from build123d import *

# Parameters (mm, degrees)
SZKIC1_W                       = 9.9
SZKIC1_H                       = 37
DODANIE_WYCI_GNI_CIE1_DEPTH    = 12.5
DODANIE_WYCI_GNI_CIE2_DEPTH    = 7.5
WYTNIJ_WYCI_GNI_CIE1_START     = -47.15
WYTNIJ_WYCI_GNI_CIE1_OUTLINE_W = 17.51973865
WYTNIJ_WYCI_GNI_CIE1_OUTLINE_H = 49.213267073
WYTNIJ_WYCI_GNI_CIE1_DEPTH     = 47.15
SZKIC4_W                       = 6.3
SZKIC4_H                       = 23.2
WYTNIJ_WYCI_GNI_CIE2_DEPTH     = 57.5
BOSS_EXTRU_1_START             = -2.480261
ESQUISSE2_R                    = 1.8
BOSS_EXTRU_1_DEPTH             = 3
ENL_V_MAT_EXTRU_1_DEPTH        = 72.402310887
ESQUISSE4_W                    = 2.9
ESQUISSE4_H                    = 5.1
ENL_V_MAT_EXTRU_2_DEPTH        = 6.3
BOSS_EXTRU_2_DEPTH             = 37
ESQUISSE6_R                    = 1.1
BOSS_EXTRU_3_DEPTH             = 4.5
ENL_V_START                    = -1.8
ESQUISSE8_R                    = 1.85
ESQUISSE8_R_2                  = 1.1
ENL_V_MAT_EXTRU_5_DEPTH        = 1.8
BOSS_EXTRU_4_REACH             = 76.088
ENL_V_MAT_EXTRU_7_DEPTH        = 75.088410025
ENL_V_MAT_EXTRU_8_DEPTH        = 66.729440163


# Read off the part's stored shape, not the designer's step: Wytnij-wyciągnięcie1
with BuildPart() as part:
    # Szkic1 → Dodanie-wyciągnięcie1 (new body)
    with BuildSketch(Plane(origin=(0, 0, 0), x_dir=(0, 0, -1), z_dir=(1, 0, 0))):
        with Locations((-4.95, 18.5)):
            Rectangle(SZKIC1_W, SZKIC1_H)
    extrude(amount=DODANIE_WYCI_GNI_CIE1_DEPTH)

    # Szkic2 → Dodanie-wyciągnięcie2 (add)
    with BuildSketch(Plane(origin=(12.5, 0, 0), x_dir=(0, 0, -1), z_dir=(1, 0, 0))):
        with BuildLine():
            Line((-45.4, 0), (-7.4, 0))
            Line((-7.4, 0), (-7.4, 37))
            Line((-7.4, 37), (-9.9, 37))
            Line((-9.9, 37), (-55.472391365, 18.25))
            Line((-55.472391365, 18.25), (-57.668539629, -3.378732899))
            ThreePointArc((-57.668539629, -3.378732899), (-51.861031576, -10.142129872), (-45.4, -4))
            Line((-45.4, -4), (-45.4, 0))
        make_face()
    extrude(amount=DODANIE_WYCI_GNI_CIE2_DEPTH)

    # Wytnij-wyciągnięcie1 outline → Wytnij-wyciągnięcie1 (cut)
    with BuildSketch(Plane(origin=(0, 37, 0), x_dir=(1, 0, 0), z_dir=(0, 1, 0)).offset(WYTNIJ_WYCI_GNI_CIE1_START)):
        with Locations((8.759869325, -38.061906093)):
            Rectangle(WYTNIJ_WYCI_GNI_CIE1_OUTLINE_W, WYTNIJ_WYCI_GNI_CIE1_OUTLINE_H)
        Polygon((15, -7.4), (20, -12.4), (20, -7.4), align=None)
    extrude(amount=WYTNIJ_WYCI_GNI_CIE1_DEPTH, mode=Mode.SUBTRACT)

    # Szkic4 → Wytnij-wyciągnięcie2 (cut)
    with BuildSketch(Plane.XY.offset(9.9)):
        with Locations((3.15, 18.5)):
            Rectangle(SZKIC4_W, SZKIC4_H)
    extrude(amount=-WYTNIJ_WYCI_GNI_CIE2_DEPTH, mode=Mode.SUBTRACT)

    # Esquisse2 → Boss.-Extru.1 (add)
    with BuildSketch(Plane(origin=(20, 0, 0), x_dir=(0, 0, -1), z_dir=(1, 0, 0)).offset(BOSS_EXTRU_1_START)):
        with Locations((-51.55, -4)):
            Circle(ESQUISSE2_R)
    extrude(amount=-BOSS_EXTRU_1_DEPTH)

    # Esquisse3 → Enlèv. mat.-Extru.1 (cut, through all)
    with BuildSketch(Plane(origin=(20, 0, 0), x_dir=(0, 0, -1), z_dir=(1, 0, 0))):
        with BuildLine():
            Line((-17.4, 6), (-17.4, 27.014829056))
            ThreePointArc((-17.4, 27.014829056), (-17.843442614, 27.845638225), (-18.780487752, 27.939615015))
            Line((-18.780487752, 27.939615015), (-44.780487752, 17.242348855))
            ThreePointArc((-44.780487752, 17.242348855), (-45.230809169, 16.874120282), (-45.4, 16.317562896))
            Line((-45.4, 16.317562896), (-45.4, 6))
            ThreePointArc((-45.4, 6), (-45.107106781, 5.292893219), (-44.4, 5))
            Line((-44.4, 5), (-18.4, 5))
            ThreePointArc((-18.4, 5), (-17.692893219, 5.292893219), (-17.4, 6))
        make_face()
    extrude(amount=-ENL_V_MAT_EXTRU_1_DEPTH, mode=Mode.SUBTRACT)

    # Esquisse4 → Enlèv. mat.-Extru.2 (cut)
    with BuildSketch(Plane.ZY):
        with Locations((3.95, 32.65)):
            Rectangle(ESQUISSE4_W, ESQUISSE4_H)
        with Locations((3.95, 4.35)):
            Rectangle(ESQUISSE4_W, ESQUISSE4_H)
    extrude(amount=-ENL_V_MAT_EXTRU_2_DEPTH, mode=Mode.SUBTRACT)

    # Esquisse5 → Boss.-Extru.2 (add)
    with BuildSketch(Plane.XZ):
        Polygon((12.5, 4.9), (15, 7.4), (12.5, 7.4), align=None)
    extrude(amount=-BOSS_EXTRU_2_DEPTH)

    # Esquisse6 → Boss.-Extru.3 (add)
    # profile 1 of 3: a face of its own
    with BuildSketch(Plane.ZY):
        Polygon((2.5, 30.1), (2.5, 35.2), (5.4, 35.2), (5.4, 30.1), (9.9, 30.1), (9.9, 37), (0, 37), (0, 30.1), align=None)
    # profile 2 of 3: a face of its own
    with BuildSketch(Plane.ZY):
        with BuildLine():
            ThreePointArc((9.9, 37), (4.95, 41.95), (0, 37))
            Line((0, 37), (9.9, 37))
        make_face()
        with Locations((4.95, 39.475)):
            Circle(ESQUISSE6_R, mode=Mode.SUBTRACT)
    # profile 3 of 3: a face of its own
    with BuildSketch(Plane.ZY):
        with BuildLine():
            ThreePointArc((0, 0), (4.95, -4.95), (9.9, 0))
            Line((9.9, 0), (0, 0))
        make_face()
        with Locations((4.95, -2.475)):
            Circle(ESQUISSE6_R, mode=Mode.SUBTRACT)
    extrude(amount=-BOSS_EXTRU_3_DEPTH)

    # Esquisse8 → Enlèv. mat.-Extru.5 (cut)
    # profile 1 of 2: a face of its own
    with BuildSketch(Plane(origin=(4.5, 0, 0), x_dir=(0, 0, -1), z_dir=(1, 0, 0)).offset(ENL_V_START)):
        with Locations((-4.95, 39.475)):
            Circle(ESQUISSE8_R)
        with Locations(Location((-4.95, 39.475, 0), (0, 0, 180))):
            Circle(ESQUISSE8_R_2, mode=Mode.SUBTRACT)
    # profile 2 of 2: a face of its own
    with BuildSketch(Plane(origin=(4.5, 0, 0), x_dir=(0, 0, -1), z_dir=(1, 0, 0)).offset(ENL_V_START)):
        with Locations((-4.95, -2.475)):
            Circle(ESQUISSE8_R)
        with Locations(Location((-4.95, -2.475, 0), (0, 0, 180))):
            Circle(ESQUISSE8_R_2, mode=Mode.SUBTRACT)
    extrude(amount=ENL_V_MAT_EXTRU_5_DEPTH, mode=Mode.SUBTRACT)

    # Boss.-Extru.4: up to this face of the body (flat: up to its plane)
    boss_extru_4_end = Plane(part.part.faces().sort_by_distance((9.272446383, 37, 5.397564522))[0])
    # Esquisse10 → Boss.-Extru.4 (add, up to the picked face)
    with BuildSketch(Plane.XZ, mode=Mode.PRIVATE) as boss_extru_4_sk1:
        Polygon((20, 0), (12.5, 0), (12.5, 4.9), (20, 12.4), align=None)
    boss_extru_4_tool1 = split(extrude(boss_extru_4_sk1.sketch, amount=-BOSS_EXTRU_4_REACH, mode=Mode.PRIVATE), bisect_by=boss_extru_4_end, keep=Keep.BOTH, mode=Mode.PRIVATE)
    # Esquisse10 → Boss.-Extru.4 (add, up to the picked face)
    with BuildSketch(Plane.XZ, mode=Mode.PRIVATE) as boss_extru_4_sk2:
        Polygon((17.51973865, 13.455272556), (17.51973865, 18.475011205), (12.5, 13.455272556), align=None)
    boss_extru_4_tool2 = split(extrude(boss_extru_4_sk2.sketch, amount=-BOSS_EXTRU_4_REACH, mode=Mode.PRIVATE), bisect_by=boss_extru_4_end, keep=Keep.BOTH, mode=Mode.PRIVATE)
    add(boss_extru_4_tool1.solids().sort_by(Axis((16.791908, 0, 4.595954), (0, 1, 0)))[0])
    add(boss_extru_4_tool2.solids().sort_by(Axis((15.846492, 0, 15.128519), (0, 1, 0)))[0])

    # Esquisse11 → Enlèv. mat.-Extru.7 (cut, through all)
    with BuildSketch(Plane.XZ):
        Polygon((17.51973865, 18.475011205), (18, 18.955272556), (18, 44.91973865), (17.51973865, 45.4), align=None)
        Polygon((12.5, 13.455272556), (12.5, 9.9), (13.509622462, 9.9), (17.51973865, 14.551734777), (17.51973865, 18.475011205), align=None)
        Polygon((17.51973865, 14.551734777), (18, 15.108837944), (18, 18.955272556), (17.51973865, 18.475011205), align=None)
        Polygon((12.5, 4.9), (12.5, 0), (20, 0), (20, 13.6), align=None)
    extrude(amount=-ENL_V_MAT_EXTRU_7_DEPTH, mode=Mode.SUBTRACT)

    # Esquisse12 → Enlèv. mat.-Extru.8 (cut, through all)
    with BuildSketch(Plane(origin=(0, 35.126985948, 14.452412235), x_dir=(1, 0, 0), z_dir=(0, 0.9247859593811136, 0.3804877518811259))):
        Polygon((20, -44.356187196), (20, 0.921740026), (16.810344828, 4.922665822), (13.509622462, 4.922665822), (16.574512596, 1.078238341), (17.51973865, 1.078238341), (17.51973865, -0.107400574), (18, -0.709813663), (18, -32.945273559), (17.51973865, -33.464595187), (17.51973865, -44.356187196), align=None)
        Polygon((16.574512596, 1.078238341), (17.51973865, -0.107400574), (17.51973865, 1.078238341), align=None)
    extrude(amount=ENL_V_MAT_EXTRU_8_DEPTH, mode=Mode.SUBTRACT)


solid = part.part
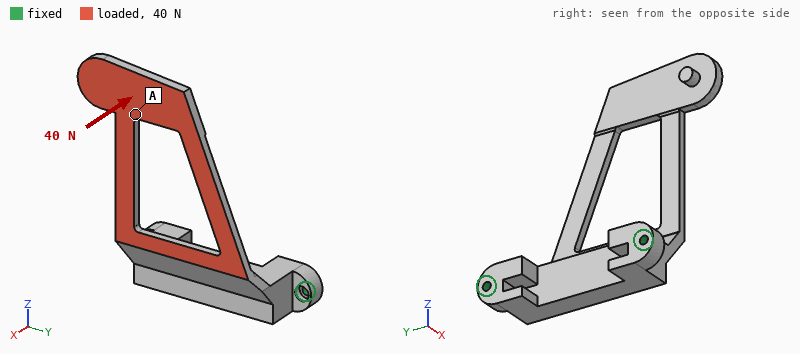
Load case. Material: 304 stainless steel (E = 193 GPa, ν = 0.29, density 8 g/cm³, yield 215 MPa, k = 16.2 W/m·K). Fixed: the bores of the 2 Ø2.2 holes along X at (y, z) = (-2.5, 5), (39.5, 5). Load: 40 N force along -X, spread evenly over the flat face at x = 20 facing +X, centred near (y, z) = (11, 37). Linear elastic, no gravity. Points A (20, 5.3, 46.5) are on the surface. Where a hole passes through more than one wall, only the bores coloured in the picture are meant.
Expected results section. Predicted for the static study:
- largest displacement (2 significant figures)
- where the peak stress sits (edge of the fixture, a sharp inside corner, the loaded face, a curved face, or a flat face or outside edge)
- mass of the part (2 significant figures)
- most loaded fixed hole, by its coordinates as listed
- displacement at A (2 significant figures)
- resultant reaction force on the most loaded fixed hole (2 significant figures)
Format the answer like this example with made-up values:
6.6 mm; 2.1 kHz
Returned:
0.46 mm; the loaded face; 46 g; (-2.5, 5); 0.30 mm; 34 N
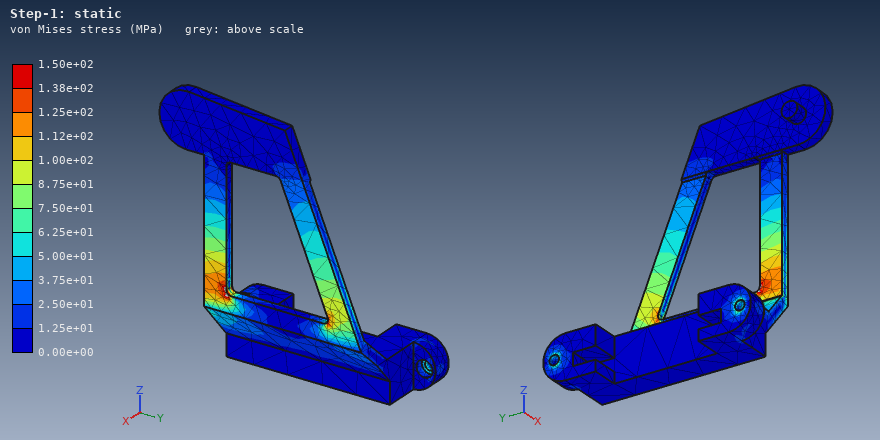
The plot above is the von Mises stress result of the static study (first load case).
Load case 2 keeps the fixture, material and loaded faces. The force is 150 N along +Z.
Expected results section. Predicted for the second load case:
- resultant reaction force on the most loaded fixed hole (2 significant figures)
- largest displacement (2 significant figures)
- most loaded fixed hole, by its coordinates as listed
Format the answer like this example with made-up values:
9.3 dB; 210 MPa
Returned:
100 N; 0.16 mm; (-2.5, 5)
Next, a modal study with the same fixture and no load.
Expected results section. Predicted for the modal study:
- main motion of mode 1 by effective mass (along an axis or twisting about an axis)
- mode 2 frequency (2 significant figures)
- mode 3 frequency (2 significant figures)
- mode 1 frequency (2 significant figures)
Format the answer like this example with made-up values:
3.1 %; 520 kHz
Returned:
along X; 1800 Hz; 2500 Hz; 460 Hz
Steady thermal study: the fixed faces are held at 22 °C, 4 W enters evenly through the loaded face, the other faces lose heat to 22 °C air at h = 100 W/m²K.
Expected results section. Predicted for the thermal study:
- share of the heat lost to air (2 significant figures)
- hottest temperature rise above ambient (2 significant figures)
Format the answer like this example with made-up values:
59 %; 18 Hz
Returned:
93 %; 32 K
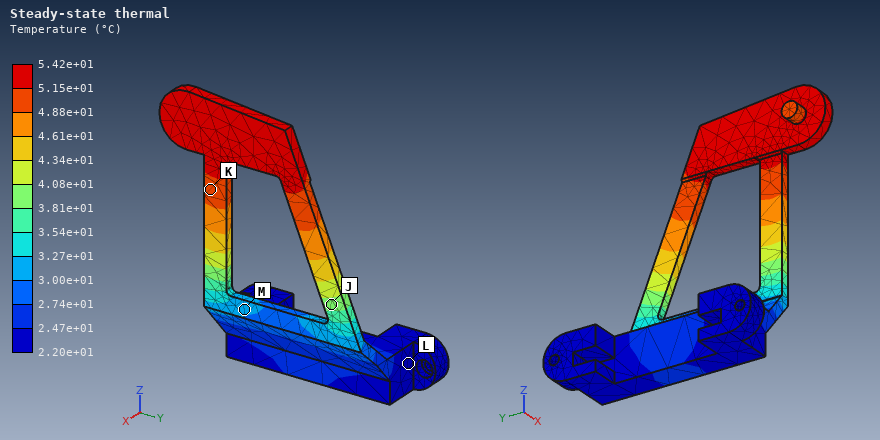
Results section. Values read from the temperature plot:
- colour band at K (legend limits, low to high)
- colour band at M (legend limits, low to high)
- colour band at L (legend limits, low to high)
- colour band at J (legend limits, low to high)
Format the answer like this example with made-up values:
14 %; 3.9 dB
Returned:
4.88e+01 to 5.15e+01 °C; 3.00e+01 to 3.27e+01 °C; 2.20e+01 to 2.47e+01 °C; 3.81e+01 to 4.08e+01 °C
